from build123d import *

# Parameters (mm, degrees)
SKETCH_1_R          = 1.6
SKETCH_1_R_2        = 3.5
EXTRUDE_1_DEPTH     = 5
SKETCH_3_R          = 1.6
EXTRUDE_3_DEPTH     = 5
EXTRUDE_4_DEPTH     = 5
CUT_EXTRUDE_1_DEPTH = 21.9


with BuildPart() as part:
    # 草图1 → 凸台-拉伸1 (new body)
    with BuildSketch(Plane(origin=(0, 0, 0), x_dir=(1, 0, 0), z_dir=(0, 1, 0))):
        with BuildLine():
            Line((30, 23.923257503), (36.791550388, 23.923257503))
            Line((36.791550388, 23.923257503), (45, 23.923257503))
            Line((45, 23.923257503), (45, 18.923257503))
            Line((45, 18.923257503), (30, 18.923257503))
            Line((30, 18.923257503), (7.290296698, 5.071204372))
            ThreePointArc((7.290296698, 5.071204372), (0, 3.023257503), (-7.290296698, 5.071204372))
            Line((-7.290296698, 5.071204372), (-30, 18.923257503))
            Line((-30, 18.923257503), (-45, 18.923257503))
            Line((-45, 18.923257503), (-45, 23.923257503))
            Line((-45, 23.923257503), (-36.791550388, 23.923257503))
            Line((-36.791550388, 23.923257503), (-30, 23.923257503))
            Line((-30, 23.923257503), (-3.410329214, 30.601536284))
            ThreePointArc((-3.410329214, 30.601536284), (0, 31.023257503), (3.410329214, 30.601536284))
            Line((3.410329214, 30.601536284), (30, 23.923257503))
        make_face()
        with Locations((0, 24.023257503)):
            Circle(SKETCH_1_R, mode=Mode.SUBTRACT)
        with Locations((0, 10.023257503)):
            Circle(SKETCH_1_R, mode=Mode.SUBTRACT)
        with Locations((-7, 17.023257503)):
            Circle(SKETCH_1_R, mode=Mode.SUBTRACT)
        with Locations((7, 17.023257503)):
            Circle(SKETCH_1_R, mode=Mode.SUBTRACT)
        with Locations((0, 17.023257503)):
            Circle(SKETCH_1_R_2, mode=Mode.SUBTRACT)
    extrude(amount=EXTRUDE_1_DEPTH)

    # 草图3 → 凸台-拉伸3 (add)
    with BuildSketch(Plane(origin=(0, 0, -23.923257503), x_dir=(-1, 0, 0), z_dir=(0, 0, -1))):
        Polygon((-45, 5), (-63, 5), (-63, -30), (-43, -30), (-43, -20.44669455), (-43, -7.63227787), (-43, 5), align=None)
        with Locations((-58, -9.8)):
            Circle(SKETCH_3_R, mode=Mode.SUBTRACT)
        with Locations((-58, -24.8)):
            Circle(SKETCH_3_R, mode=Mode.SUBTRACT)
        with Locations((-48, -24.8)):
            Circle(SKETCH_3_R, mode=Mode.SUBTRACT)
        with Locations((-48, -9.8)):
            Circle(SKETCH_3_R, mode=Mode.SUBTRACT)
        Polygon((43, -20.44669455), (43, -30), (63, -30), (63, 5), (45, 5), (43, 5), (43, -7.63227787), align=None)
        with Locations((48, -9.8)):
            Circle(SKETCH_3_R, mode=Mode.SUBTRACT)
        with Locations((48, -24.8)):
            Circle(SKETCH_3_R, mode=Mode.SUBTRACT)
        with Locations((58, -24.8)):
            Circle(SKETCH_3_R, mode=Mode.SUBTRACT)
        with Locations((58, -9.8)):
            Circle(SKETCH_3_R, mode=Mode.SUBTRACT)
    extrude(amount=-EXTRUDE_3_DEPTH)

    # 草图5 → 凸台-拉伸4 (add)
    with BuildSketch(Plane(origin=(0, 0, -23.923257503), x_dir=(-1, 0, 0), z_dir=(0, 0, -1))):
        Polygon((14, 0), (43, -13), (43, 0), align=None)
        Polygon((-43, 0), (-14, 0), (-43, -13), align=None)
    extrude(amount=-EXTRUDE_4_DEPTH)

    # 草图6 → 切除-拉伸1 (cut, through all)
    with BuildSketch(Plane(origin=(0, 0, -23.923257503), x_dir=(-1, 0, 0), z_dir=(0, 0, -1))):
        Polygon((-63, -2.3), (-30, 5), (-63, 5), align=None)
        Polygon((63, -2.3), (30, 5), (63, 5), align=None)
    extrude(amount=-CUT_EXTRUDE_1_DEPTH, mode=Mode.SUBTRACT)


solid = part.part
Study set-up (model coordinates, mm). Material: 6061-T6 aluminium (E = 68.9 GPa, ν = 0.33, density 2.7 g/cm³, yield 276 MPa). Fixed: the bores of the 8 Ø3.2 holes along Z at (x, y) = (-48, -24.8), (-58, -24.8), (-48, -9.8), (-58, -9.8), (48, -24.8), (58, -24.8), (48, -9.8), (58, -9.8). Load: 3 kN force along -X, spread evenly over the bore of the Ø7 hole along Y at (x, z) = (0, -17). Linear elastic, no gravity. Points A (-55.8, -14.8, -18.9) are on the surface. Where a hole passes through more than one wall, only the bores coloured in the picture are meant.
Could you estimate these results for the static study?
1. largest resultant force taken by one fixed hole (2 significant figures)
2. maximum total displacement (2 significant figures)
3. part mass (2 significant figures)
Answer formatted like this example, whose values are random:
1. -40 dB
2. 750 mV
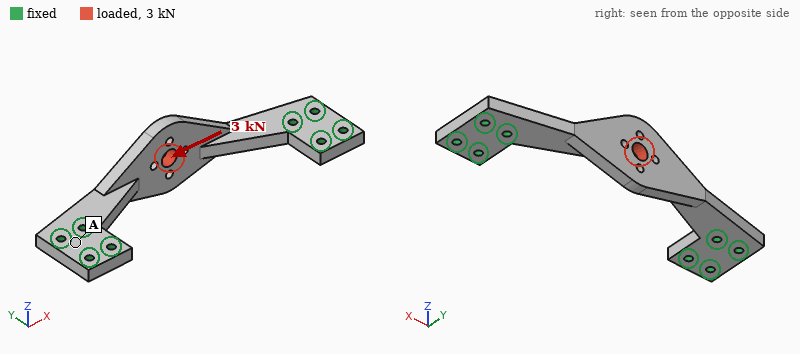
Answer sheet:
1. 1.1 kN
2. 50 µm
3. 35 g
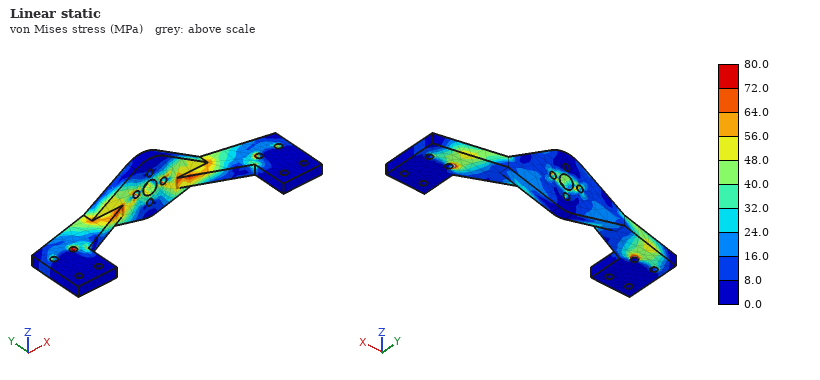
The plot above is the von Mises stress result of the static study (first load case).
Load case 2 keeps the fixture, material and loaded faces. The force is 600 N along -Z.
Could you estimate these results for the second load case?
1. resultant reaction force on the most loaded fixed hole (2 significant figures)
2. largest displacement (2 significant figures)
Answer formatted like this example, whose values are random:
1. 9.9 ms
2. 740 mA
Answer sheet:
1. 480 N
2. 0.13 mm
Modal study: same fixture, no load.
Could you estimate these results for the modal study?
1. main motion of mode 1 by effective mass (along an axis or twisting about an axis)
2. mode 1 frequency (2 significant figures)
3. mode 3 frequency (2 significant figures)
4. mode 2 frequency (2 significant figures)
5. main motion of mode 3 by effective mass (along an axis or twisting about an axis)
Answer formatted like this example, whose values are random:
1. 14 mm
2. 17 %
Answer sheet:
1. along Z
2. 3100 Hz
3. 7100 Hz
4. 4900 Hz
5. along Y
